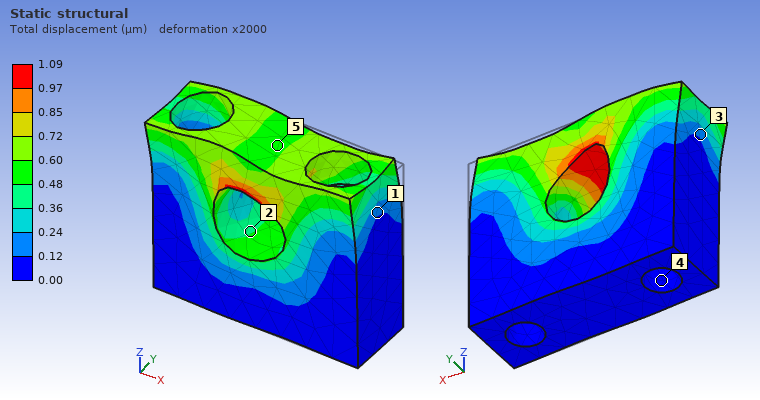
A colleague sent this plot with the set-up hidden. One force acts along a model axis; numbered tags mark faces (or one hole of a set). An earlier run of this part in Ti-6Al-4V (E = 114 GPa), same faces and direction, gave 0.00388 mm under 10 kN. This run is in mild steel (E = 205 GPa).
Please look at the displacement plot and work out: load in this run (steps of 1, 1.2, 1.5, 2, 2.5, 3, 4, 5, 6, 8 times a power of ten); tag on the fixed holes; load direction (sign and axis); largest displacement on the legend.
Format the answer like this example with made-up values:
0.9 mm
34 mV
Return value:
5 kN
4
-X
1.09 µm
